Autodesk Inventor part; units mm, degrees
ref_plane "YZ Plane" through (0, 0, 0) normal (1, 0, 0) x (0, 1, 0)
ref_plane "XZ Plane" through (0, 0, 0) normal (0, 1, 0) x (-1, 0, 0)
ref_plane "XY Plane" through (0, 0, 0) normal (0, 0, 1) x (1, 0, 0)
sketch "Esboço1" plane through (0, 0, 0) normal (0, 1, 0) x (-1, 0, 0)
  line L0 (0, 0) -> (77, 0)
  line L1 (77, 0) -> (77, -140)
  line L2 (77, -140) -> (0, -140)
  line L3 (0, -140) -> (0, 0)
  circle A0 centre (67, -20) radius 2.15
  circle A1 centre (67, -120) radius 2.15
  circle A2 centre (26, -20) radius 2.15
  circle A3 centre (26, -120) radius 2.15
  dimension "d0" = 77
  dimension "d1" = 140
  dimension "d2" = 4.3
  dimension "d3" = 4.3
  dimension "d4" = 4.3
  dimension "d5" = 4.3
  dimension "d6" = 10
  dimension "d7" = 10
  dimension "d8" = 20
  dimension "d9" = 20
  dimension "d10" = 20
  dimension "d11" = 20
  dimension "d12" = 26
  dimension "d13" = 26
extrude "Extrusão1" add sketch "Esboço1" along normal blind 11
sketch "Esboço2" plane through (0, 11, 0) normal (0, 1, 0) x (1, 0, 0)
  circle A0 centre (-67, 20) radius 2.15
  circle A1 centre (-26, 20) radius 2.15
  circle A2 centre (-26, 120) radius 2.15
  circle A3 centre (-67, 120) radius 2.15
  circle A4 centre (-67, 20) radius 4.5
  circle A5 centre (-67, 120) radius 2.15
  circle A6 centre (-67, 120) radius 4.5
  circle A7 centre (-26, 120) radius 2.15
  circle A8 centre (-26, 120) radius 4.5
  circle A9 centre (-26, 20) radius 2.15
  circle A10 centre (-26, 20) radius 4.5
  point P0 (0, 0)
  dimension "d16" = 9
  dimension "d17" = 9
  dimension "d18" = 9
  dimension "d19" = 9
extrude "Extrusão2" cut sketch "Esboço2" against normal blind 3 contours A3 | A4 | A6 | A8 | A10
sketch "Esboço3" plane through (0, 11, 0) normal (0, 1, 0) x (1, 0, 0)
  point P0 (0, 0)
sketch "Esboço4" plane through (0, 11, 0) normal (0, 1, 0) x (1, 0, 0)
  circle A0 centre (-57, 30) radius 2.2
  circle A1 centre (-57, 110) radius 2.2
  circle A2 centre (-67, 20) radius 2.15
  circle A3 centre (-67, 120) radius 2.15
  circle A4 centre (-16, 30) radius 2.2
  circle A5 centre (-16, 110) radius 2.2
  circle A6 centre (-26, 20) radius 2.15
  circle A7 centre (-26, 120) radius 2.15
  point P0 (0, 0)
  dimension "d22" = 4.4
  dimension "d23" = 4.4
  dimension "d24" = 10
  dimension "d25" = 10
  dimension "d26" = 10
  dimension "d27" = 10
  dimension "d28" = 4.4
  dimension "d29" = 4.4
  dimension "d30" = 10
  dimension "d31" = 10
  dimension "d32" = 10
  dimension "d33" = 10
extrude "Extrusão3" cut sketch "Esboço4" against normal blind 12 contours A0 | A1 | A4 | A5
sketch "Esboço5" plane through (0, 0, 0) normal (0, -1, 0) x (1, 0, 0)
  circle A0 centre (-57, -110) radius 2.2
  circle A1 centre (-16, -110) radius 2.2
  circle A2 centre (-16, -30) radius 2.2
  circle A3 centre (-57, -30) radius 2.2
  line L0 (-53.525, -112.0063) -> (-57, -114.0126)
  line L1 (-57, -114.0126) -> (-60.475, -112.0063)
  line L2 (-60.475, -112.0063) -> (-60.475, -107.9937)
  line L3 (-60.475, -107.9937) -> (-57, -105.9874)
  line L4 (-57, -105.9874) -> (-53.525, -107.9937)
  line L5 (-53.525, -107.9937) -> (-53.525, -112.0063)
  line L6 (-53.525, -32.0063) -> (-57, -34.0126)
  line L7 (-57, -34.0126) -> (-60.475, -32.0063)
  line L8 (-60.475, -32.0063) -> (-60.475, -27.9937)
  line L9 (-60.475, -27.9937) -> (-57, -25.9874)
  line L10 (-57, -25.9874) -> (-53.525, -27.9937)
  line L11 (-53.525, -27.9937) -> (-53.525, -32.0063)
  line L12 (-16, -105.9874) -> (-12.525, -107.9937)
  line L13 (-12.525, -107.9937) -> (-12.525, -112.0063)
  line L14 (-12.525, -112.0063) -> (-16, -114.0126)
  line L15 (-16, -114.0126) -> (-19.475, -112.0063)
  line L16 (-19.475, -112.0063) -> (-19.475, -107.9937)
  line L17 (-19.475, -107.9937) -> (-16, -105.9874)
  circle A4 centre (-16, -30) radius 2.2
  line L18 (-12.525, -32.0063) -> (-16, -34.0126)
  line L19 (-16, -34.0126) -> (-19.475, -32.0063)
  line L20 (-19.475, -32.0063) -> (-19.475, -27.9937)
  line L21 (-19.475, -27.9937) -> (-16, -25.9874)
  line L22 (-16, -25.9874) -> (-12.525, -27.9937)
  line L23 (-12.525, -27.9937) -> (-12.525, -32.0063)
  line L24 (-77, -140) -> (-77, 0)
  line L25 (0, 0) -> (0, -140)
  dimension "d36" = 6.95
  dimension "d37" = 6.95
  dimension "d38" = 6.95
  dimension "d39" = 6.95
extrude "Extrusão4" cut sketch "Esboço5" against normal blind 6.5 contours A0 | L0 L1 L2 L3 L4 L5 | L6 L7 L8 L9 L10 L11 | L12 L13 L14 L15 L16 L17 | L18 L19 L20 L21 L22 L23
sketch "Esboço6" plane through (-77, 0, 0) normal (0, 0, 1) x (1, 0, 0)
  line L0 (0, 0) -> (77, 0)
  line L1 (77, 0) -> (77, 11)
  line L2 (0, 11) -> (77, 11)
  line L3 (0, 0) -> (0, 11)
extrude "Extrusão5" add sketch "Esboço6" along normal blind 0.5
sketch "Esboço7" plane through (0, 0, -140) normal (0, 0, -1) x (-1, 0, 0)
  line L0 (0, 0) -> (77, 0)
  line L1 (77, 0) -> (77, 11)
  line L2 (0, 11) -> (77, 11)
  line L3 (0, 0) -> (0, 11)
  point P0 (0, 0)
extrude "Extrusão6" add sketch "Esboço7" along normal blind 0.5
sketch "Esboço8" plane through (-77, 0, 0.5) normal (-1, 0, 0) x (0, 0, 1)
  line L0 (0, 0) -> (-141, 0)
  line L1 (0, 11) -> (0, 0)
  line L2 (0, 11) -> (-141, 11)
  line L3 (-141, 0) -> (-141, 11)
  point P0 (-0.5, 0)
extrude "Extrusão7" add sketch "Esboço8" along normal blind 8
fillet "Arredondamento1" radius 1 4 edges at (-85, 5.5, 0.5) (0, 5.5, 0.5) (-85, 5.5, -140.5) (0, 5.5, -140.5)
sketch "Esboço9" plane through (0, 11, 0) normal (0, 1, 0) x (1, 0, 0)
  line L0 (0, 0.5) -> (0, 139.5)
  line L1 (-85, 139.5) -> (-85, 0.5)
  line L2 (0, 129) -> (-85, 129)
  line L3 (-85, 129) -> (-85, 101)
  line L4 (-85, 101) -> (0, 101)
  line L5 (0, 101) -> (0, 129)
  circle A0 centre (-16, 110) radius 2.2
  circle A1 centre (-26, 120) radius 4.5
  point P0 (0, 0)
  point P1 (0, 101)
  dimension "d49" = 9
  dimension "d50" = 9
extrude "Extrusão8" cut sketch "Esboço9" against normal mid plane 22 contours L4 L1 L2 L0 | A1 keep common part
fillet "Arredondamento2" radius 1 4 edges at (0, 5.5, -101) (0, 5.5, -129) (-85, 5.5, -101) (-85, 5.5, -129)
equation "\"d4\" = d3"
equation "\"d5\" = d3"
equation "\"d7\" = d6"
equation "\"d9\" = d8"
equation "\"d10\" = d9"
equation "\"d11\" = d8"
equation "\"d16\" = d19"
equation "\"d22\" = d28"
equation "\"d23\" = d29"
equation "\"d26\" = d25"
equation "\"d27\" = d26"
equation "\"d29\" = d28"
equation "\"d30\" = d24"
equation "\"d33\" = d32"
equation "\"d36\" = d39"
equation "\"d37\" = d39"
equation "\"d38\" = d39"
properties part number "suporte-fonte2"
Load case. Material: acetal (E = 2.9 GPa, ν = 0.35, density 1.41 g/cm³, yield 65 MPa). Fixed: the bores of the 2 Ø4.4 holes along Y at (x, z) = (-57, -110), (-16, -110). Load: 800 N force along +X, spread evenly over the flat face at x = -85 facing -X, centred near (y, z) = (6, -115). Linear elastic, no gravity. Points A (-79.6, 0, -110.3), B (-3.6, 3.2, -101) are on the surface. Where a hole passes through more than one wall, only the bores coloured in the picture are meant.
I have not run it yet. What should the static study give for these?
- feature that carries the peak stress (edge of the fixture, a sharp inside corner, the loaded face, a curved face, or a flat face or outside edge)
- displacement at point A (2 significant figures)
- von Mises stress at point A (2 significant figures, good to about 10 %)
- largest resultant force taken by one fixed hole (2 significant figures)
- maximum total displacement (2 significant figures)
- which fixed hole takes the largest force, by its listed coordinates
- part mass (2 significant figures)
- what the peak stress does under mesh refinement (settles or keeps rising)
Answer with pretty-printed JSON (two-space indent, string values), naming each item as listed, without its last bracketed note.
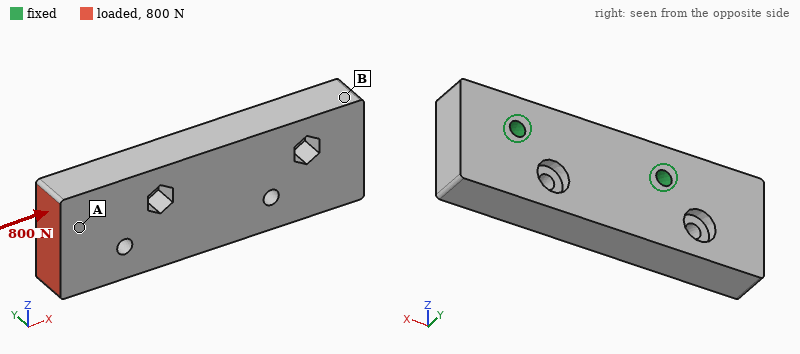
{
  "feature that carries the peak stress": "edge of the fixture",
  "displacement at point A": "78 µm",
  "von Mises stress at point A": "2.8 MPa",
  "largest resultant force taken by one fixed hole": "560 N",
  "maximum total displacement": "94 µm",
  "which fixed hole takes the largest force, by its listed coordinates": "(-57, -110)",
  "part mass": "35 g",
  "what the peak stress does under mesh refinement": "keeps rising"
}
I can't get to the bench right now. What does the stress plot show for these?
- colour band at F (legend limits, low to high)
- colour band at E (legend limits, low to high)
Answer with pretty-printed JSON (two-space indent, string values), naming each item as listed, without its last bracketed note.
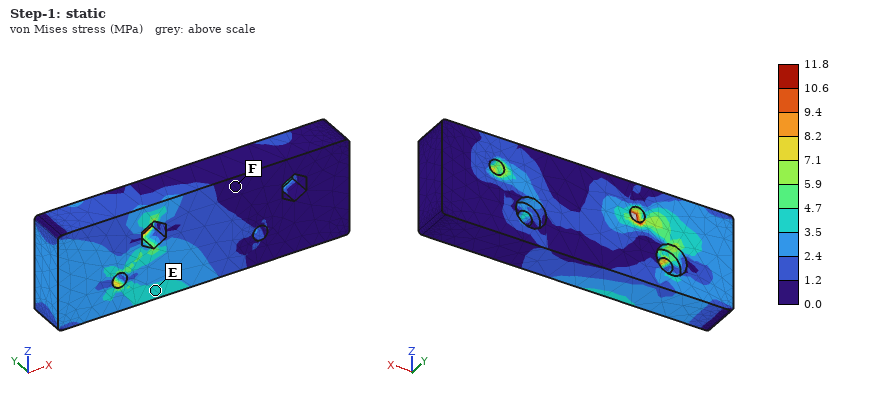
{
  "colour band at F": "0.0 to 1.2 MPa",
  "colour band at E": "3.5 to 4.7 MPa"
}
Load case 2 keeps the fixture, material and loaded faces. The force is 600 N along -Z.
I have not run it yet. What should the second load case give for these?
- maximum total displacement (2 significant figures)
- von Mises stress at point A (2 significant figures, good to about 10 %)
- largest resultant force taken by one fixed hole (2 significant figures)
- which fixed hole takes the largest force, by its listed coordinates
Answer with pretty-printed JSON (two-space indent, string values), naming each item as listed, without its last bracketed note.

{
  "maximum total displacement": "0.45 mm",
  "von Mises stress at point A": "4.4 MPa",
  "largest resultant force taken by one fixed hole": "970 N",
  "which fixed hole takes the largest force, by its listed coordinates": "(-57, -110)"
}
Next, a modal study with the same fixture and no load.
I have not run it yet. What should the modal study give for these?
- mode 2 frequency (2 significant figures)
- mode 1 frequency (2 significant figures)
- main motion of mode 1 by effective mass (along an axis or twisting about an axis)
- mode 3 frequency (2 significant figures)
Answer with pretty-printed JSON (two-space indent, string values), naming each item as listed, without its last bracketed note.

{
  "mode 2 frequency": "2000 Hz",
  "mode 1 frequency": "1600 Hz",
  "main motion of mode 1 by effective mass": "along Y",
  "mode 3 frequency": "2800 Hz"
}
